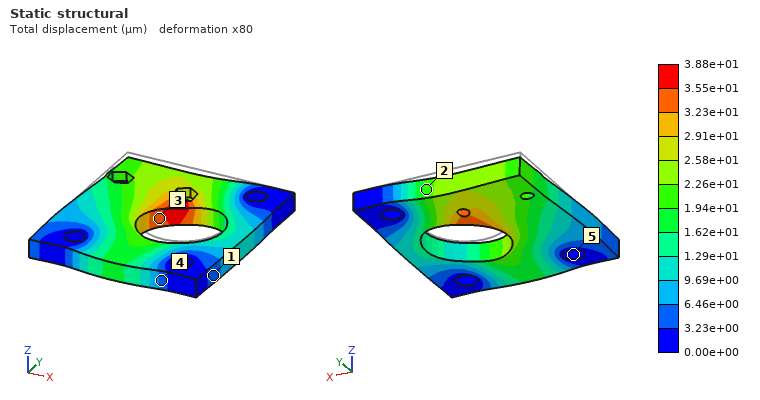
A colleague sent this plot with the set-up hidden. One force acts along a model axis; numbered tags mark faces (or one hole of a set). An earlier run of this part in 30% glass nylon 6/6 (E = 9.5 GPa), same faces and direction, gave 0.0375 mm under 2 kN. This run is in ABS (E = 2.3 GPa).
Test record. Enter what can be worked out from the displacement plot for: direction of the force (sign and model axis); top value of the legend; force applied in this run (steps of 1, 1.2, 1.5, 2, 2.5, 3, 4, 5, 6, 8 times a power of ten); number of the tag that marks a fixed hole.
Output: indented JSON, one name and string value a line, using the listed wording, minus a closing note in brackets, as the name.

{
  "direction of the force": "-Y",
  "top value of the legend": "3.88e+01 µm",
  "force applied in this run": "500 N",
  "number of the tag that marks a fixed hole": "5"
}
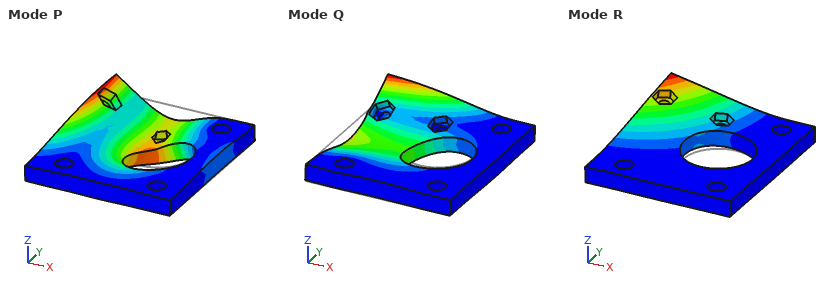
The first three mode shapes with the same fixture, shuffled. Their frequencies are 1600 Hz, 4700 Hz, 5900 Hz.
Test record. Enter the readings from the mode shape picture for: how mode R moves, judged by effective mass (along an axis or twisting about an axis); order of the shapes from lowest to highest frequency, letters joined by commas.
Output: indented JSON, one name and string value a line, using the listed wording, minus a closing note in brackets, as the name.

{
  "how mode R moves, judged by effective mass": "along Z",
  "order of the shapes from lowest to highest frequency, letters joined by commas": "R, Q, P"
}
